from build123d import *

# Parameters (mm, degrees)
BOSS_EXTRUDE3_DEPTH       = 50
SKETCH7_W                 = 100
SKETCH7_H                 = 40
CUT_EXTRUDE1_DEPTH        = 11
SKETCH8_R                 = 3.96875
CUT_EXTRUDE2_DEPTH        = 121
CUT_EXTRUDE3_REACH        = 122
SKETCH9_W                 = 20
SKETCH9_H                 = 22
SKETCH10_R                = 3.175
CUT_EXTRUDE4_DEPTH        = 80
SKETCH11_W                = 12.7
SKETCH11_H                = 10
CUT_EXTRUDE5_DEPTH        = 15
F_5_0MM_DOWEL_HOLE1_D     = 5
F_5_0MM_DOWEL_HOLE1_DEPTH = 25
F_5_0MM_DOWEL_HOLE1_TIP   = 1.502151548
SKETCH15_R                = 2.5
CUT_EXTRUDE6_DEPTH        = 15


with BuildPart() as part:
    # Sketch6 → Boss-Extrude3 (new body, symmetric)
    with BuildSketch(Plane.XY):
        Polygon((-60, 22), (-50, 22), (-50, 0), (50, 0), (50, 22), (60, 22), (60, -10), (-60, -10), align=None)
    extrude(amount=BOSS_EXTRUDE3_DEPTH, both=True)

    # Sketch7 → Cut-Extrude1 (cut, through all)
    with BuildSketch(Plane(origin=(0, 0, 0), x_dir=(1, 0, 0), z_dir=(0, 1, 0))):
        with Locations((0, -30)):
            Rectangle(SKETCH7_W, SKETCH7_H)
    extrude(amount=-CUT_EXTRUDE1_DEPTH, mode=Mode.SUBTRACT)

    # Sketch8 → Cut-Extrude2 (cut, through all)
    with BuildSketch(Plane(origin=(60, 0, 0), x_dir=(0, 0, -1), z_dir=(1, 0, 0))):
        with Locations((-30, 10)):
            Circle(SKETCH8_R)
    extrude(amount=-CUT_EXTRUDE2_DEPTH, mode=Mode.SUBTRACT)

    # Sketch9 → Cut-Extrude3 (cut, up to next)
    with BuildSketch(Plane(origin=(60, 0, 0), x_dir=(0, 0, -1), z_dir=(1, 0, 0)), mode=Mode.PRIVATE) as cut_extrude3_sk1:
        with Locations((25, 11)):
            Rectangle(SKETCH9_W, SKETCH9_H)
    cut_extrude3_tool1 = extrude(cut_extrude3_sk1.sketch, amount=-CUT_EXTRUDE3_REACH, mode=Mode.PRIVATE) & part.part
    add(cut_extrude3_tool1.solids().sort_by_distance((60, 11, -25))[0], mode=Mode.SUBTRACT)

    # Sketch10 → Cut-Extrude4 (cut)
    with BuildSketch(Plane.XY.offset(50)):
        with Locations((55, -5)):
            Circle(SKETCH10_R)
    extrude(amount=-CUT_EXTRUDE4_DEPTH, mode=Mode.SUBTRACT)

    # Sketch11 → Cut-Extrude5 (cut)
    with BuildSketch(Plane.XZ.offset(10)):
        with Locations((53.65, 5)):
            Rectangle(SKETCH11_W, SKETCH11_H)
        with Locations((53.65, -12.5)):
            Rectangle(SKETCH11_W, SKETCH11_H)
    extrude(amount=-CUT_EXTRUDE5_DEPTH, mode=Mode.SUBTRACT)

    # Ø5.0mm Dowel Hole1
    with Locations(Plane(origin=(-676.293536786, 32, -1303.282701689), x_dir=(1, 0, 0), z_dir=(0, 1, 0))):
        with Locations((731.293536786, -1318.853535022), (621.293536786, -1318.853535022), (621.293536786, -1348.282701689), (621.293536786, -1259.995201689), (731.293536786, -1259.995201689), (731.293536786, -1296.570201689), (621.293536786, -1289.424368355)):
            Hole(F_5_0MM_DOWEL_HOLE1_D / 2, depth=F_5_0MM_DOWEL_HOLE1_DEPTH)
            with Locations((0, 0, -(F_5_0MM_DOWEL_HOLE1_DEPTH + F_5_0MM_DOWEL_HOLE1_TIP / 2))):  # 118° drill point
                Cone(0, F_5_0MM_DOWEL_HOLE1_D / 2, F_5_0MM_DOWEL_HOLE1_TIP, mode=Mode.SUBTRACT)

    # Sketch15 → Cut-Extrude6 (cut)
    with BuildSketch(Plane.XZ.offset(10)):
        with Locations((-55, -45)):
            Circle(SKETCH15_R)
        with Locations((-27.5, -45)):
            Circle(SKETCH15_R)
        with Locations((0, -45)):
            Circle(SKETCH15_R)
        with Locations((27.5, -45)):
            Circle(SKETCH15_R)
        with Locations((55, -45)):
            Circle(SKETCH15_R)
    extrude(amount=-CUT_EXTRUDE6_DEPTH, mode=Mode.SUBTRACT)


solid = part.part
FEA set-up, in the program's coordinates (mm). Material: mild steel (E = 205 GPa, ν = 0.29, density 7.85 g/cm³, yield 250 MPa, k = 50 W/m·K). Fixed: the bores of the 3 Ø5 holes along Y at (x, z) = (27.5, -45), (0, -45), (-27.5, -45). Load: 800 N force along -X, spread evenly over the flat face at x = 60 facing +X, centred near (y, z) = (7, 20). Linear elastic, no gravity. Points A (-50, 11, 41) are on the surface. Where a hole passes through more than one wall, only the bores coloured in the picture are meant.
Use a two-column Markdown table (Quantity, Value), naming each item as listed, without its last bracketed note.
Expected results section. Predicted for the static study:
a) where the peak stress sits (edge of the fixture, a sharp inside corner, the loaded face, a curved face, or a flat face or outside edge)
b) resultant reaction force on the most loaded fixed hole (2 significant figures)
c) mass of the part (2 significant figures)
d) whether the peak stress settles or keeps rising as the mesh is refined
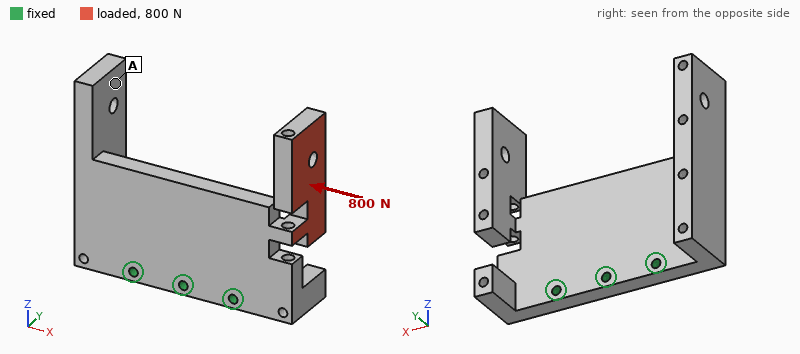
| Quantity | Value |
|---|---|
| where the peak stress sits | a sharp inside corner |
| resultant reaction force on the most loaded fixed hole | 970 N |
| mass of the part | 860 g |
| whether the peak stress settles or keeps rising as the mesh is refined | keeps rising |
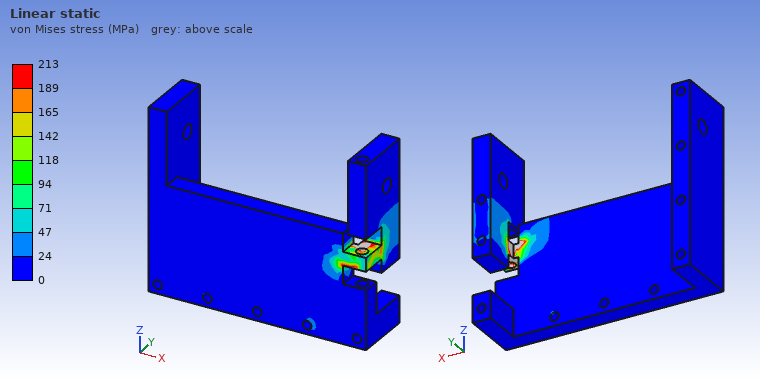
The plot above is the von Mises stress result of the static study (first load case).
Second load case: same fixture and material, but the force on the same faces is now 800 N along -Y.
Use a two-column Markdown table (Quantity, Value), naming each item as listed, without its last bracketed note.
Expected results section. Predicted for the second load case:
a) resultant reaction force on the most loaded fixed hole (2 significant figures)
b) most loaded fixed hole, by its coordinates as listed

| Quantity | Value |
|---|---|
| resultant reaction force on the most loaded fixed hole | 1.1 kN |
| most loaded fixed hole, by its coordinates as listed | (27.5, -45) |
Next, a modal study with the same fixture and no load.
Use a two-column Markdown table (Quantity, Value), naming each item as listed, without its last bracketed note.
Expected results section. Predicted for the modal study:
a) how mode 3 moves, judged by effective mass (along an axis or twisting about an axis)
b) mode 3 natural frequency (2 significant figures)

| Quantity | Value |
|---|---|
| how mode 3 moves, judged by effective mass | along Y |
| mode 3 natural frequency | 1000 Hz |
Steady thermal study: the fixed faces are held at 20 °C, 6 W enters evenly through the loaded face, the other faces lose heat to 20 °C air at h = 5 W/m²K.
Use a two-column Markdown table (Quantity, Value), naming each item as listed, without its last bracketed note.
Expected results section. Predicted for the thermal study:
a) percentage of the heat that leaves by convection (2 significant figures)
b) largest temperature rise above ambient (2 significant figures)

| Quantity | Value |
|---|---|
| percentage of the heat that leaves by convection | 25 % |
| largest temperature rise above ambient | 51 K |
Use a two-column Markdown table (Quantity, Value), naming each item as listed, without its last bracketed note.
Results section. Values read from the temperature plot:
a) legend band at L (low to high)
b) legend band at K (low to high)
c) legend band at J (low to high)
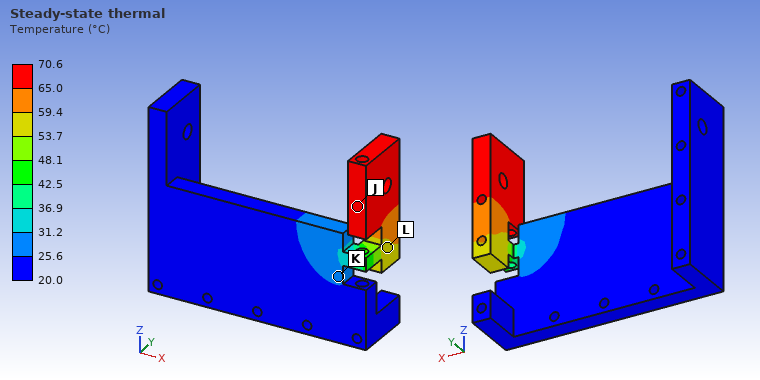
| Quantity | Value |
|---|---|
| legend band at L | 53.7 to 59.4 °C |
| legend band at K | 25.6 to 31.2 °C |
| legend band at J | 65.0 to 70.6 °C |
